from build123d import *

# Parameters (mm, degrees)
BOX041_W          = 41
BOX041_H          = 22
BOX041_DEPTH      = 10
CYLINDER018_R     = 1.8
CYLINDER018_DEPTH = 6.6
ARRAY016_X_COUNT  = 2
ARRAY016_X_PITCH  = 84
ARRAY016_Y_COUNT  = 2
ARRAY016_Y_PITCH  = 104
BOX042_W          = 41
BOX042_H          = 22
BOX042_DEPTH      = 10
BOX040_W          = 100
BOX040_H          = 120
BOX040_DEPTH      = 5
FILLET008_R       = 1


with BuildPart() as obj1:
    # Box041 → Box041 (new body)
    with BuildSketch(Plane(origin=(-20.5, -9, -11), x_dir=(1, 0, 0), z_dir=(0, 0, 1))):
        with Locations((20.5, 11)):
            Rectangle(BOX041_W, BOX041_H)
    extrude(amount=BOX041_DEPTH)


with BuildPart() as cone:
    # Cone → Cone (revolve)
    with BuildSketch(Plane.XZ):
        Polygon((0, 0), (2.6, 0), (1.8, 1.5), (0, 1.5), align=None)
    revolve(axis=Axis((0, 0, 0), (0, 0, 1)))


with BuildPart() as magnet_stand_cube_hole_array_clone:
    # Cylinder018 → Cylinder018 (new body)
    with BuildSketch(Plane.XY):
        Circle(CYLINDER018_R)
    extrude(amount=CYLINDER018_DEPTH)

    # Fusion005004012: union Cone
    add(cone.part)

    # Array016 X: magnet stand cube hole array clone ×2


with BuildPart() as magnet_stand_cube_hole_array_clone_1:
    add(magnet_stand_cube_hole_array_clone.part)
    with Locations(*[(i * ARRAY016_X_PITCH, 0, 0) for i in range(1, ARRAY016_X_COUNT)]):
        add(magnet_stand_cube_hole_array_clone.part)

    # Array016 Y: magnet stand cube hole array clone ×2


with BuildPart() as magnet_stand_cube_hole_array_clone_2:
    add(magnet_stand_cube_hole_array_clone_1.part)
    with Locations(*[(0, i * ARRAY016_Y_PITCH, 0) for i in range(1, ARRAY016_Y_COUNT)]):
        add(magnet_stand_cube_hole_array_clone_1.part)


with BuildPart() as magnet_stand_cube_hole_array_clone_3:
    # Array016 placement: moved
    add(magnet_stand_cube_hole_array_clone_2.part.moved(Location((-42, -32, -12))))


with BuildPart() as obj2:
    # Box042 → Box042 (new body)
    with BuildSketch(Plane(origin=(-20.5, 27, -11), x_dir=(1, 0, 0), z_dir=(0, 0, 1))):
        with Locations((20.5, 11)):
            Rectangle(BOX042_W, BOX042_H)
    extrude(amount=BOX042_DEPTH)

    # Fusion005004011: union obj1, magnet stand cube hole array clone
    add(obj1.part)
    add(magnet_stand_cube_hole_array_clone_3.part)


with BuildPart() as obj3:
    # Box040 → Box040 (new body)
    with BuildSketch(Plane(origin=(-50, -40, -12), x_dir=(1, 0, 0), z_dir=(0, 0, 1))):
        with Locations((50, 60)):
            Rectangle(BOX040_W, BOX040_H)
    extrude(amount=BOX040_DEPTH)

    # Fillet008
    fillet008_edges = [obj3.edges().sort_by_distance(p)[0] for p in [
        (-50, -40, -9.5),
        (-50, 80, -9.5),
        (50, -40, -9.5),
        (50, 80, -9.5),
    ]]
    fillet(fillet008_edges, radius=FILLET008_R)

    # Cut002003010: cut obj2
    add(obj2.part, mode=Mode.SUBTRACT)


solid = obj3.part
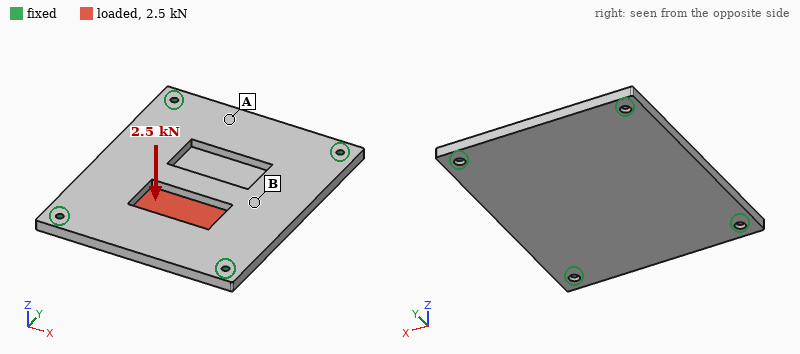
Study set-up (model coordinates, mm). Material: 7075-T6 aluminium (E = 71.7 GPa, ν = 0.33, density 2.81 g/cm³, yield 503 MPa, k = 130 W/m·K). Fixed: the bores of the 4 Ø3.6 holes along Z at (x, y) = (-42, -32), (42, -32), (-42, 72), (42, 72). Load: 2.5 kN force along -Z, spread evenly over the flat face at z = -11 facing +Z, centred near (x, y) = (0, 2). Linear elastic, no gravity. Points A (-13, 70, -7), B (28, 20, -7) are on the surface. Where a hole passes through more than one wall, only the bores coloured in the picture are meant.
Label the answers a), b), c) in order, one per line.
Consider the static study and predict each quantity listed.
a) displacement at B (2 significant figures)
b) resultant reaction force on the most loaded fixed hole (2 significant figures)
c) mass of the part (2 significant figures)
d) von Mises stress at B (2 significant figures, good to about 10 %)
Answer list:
a) 0.37 mm
b) 1.7 kN
c) 150 g
d) 73 MPa
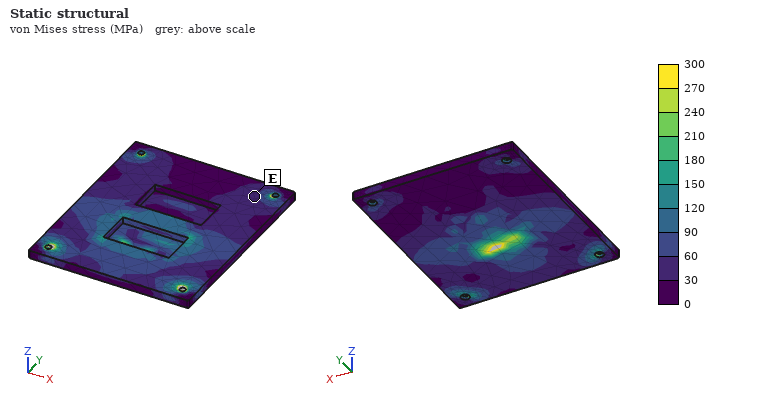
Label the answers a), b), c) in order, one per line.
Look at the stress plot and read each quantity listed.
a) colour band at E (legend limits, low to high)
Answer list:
a) 30 to 60 MPa
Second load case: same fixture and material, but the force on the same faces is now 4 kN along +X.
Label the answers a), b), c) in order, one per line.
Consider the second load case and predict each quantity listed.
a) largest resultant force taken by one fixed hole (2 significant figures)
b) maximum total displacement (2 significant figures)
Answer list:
a) 1.5 kN
b) 20 µm
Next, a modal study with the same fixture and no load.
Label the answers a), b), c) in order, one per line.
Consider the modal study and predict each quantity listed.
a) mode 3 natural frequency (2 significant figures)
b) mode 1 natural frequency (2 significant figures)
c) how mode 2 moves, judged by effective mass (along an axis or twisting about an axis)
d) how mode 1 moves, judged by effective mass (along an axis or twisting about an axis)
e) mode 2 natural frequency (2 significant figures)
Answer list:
a) 3200 Hz
b) 1700 Hz
c) twisting about Y
d) along Z
e) 2500 Hz
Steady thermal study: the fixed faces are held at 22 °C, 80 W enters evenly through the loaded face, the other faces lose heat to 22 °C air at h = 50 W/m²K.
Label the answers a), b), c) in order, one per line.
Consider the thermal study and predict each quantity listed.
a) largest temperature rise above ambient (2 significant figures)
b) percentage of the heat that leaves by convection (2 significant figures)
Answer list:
a) 80 K
b) 33 %
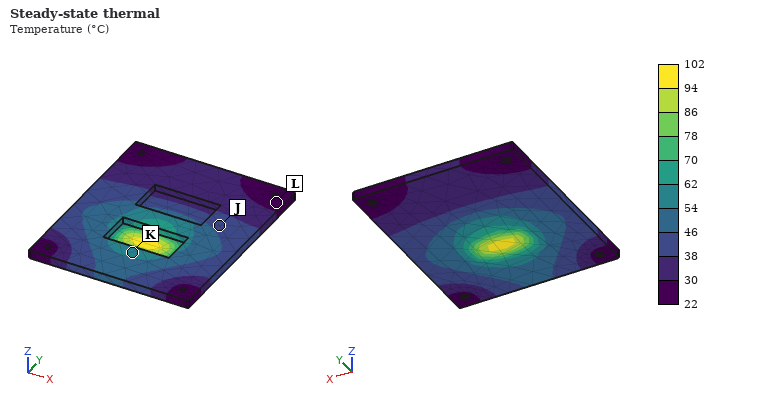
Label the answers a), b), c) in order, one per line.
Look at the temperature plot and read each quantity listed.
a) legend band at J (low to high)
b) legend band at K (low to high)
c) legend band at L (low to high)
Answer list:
a) 38 to 46 °C
b) 54 to 62 °C
c) 22 to 30 °C
